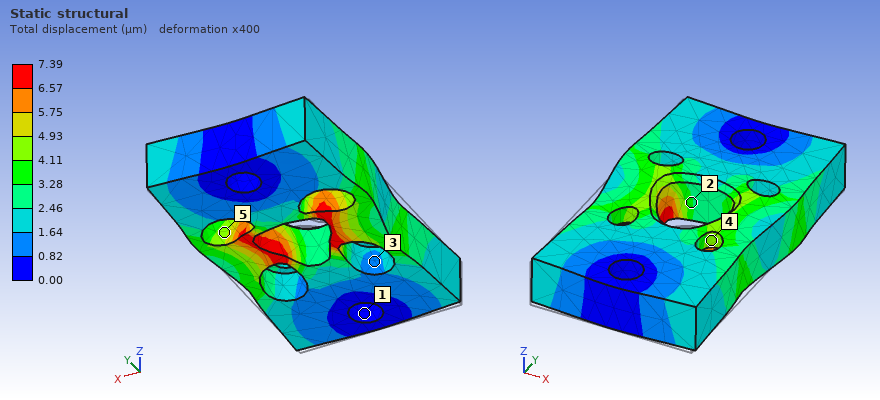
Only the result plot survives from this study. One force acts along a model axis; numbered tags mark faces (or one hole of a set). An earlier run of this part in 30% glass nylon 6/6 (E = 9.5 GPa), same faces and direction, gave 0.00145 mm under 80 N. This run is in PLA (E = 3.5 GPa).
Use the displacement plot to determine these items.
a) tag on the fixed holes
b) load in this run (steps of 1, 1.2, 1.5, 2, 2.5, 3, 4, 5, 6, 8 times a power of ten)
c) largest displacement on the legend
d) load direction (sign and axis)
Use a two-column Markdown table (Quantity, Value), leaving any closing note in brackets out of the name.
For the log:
| Quantity | Value |
|---|---|
| tag on the fixed holes | 1 |
| load in this run | 150 N |
| largest displacement on the legend | 7.39 µm |
| load direction | +Y |
